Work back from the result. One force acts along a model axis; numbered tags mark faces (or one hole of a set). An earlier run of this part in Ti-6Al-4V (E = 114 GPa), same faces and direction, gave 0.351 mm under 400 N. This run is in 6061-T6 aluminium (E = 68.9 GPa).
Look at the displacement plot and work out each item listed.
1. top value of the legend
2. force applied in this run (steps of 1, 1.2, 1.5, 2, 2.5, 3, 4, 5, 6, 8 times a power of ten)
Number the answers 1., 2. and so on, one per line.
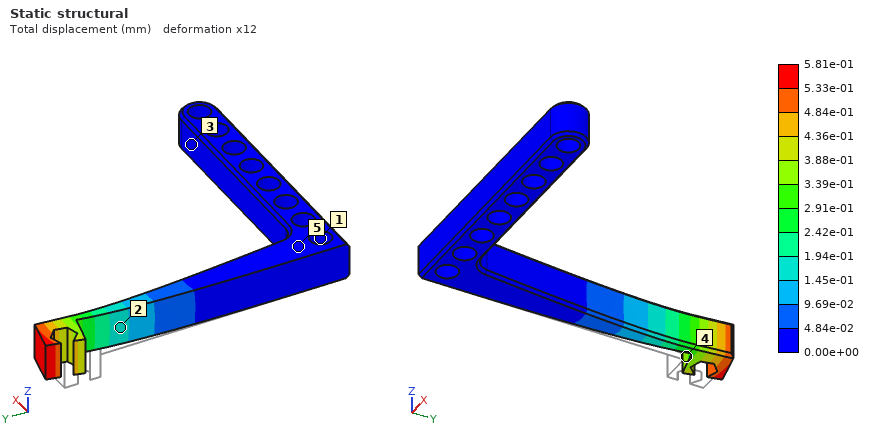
1. 5.81e-01 mm
2. 400 N
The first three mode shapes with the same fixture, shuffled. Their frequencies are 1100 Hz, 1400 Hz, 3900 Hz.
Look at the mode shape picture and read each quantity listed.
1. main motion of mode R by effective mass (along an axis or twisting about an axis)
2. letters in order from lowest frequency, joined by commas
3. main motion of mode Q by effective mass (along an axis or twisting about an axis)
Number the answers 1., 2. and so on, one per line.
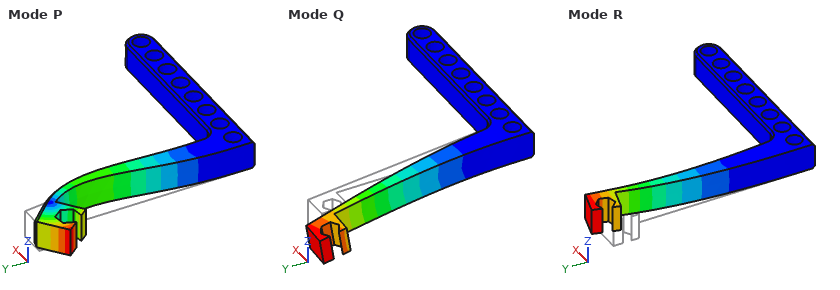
1. along X
2. R, Q, P
3. along Z
